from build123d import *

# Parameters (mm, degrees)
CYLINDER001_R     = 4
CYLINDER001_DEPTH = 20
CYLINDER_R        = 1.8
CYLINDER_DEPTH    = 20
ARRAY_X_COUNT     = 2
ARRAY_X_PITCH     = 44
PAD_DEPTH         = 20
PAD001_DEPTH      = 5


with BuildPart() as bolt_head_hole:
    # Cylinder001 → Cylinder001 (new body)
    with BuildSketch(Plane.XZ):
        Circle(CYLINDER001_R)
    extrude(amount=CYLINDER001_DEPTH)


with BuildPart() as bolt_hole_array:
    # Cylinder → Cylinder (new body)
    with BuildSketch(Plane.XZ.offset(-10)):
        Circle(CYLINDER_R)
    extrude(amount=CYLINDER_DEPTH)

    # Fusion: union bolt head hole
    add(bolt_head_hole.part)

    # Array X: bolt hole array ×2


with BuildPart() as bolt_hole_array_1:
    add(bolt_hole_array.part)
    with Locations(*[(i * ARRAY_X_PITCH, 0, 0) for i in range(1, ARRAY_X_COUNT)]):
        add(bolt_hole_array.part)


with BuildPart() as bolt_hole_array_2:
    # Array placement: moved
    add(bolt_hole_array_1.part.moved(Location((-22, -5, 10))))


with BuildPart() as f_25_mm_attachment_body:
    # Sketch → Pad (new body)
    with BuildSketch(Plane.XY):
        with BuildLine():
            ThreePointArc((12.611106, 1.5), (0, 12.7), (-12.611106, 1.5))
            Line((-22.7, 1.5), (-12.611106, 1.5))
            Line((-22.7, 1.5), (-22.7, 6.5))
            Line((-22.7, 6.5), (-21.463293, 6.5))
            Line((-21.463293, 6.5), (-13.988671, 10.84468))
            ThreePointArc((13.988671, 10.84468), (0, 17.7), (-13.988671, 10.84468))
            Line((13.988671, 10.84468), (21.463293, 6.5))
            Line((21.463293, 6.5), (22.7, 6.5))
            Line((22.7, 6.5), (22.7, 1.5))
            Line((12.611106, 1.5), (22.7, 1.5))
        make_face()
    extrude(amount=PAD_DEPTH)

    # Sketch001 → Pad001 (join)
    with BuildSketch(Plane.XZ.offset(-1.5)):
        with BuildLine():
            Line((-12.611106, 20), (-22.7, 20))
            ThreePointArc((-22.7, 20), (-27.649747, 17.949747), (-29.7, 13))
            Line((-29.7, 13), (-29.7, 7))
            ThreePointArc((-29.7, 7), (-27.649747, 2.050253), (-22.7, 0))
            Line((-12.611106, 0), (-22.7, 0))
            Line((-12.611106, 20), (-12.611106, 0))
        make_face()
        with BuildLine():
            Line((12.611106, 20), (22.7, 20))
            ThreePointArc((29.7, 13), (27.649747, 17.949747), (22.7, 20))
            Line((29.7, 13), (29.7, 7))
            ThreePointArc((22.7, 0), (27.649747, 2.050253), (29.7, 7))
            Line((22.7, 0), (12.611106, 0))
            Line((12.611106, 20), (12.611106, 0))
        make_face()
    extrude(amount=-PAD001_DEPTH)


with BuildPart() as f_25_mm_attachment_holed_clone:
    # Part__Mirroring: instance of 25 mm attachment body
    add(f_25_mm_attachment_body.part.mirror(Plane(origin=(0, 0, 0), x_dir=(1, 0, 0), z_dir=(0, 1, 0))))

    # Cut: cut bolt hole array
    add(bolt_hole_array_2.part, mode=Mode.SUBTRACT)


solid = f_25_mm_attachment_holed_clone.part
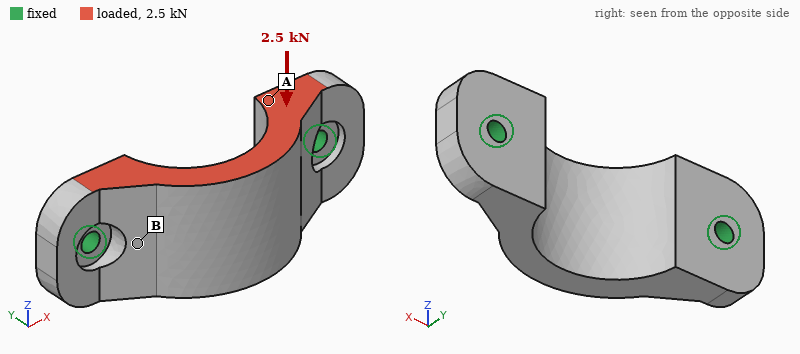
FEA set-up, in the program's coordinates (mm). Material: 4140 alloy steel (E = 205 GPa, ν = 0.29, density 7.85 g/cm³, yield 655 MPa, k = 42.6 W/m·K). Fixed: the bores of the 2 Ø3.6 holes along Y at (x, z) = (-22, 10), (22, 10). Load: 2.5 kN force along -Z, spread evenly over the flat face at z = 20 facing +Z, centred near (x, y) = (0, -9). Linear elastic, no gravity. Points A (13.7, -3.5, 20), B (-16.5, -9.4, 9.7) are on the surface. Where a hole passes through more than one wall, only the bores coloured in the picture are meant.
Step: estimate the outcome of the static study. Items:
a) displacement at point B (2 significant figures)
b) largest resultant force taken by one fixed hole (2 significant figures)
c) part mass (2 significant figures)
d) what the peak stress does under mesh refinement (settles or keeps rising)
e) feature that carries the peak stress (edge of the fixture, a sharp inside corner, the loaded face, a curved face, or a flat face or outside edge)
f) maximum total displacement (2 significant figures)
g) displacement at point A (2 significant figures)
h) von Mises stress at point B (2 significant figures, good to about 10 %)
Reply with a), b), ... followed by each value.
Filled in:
a) 12 µm
b) 1.3 kN
c) 54 g
d) keeps rising
e) edge of the fixture
f) 34 µm
g) 15 µm
h) 71 MPa
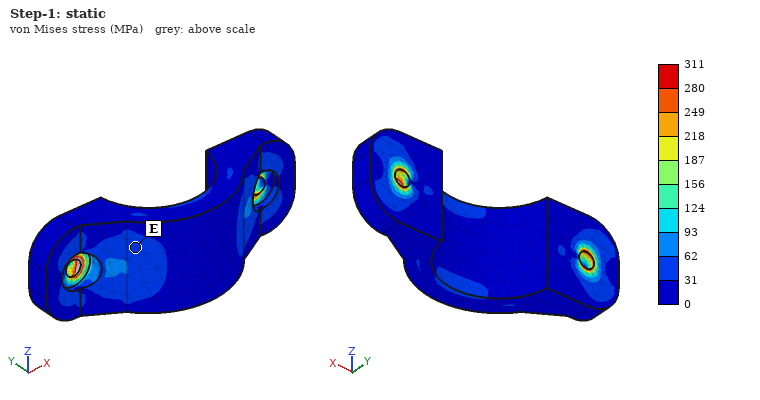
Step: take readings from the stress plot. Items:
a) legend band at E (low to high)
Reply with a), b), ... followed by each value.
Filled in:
a) 31 to 62 MPa
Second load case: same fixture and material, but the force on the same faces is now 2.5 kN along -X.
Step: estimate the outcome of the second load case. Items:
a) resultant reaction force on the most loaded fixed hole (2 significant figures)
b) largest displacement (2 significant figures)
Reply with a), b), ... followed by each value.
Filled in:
a) 1.4 kN
b) 8.9 µm
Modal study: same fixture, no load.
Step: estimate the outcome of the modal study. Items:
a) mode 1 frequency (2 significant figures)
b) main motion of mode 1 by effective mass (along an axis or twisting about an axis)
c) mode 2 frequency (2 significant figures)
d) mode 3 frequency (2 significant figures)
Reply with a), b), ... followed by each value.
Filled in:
a) 7300 Hz
b) along Z
c) 19 kHz
d) 19 kHz
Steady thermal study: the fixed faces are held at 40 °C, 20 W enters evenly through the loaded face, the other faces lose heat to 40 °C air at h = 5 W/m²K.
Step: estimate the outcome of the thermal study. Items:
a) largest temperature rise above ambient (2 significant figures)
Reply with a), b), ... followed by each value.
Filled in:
a) 44 K
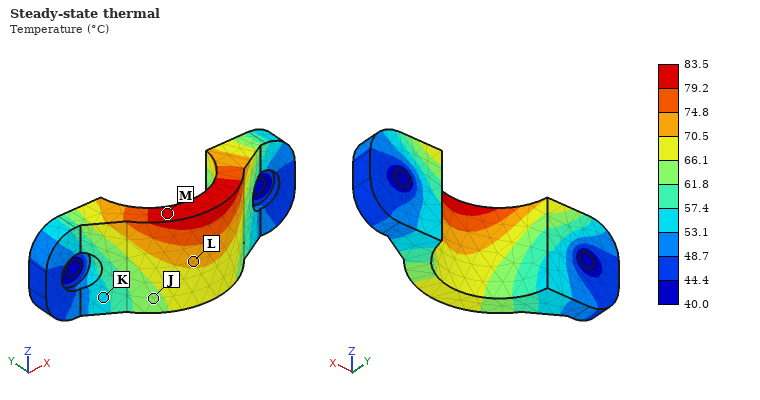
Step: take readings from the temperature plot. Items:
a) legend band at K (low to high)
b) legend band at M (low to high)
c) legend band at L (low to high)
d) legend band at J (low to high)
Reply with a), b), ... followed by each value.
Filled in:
a) 53.1 to 57.4 °C
b) 79.2 to 83.5 °C
c) 70.5 to 74.8 °C
d) 61.8 to 66.1 °C
